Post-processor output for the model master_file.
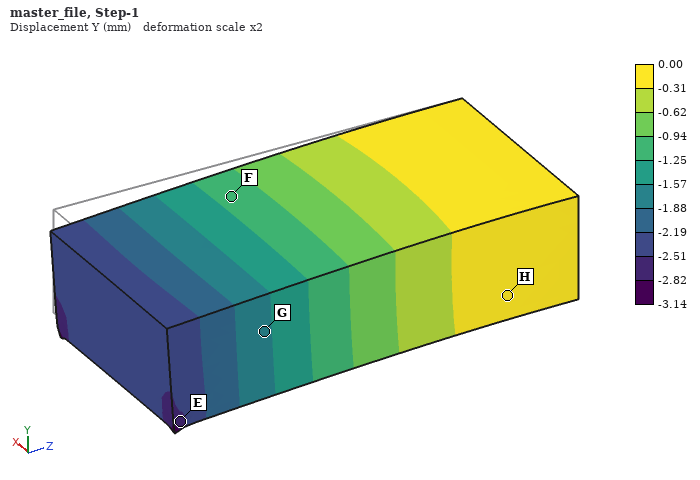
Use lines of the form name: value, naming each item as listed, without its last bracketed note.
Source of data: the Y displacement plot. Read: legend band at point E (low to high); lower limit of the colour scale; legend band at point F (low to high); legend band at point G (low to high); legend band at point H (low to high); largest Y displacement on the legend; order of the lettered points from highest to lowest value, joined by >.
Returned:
legend band at point E: -2.82 to -2.51 mm
lower limit of the colour scale: -3.14 mm
legend band at point F: -1.25 to -0.94 mm
legend band at point G: -1.88 to -1.57 mm
legend band at point H: -0.31 to 0.00 mm
largest Y displacement on the legend: 0.00 mm
order of the lettered points from highest to lowest value, joined by >: H > F > G > E
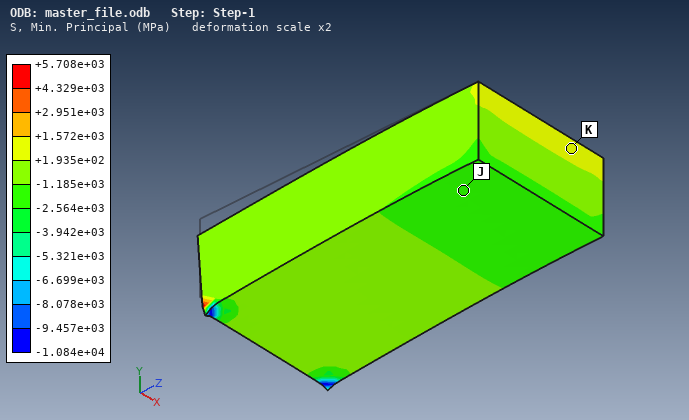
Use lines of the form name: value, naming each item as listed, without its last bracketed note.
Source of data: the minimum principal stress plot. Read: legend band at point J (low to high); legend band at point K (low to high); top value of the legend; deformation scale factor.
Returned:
legend band at point J: -2.564e+03 to -1.185e+03 MPa
legend band at point K: +1.935e+02 to +1.572e+03 MPa
top value of the legend: +5.708e+03 MPa
deformation scale factor: 2
